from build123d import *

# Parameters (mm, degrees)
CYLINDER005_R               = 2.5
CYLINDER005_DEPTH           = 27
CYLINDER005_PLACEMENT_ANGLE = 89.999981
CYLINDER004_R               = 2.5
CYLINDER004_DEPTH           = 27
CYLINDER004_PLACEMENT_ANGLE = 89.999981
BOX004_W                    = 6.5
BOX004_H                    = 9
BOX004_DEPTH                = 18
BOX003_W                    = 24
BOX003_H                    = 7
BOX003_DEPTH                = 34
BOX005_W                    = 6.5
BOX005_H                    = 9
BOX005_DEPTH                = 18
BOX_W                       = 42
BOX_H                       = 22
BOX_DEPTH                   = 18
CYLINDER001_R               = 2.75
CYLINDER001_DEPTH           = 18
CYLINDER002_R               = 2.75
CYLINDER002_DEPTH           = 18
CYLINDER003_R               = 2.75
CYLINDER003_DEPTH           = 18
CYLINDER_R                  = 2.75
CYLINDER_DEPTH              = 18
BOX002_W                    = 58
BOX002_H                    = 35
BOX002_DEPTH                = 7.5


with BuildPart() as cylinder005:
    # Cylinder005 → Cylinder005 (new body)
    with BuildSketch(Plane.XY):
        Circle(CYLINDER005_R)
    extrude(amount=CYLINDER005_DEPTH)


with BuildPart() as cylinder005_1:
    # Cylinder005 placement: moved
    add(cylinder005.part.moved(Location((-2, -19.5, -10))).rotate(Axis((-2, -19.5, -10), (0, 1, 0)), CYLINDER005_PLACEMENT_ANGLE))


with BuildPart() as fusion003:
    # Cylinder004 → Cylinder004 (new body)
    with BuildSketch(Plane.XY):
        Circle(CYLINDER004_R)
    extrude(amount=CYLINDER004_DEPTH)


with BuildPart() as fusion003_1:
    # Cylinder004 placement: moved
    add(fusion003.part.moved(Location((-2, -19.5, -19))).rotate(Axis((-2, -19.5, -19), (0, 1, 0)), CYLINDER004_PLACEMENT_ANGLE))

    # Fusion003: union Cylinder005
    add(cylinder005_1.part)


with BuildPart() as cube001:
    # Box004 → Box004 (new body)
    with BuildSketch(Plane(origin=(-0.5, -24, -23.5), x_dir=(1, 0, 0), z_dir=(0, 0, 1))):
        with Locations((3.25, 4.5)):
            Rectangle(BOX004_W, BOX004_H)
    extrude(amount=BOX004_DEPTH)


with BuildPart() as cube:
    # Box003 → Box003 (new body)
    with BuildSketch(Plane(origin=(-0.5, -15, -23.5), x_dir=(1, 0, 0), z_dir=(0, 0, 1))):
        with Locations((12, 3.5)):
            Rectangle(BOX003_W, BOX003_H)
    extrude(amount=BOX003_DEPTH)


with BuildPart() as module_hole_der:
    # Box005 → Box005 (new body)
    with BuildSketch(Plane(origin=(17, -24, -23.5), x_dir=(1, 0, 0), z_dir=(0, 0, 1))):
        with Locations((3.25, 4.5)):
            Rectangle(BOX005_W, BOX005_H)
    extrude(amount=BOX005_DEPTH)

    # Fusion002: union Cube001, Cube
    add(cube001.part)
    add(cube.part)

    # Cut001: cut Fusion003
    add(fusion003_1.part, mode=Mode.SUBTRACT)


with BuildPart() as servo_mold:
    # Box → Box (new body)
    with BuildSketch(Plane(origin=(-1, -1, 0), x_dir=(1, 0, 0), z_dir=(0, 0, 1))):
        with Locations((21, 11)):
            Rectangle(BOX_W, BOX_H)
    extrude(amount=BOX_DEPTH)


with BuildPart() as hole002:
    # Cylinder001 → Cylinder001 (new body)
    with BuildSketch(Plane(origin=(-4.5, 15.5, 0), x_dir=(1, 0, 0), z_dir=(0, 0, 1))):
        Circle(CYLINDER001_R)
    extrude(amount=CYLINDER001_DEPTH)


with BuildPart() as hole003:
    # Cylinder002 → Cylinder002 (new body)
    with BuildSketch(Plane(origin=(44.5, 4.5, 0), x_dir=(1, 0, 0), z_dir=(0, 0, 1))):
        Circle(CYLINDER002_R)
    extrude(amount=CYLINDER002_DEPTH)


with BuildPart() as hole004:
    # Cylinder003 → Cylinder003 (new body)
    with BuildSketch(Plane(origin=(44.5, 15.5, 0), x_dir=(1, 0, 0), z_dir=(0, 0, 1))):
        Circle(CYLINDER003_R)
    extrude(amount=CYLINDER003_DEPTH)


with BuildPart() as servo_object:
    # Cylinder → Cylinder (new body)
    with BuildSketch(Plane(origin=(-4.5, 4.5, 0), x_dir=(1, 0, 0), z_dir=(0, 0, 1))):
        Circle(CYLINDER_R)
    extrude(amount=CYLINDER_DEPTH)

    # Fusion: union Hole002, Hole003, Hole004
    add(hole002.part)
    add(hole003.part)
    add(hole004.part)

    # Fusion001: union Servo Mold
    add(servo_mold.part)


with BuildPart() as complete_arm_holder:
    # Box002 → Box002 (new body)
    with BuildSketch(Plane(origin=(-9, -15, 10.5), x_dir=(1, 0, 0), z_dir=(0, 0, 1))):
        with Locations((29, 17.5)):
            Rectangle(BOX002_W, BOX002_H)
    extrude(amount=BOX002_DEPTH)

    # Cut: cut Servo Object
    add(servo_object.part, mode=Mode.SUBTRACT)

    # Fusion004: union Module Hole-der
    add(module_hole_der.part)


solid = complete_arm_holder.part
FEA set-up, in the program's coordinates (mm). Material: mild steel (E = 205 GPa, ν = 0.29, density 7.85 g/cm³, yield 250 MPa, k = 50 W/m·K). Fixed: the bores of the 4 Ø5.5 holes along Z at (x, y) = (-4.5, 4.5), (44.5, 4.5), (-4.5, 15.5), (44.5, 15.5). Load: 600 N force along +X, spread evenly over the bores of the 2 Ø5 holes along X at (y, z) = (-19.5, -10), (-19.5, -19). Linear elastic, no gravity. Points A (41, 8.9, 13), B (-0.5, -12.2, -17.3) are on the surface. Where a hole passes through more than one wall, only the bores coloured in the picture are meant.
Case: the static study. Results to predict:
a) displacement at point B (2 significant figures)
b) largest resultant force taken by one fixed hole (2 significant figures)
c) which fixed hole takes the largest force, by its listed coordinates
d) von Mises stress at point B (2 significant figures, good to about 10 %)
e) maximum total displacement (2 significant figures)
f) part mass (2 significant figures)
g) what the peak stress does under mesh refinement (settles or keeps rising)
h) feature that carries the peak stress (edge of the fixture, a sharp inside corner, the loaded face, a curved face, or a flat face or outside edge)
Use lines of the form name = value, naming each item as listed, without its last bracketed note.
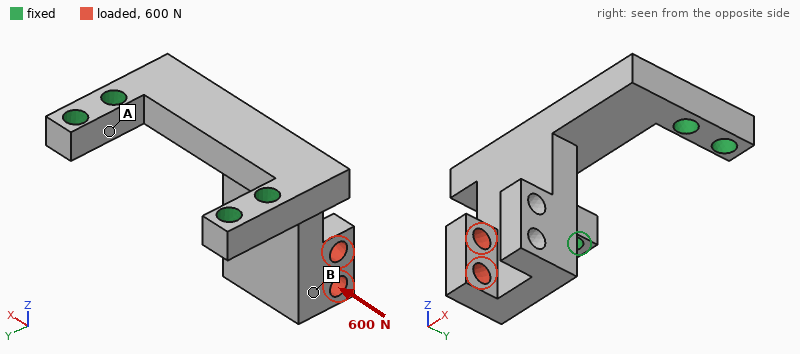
displacement at point B = 19 µm
largest resultant force taken by one fixed hole = 570 N
which fixed hole takes the largest force, by its listed coordinates = (44.5, 4.5)
von Mises stress at point B = 10 MPa
maximum total displacement = 31 µm
part mass = 120 g
what the peak stress does under mesh refinement = keeps rising
feature that carries the peak stress = edge of the fixture
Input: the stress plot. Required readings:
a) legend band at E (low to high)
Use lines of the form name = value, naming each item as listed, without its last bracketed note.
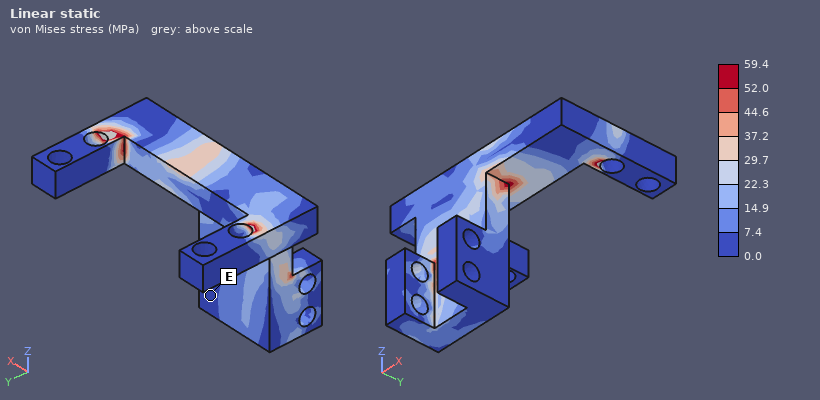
legend band at E = 0.0 to 7.4 MPa
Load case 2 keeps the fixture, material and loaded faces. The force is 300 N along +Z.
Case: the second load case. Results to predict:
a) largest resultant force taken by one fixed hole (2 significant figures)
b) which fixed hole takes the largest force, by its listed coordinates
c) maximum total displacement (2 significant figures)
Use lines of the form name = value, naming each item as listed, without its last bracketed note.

largest resultant force taken by one fixed hole = 260 N
which fixed hole takes the largest force, by its listed coordinates = (-4.5, 4.5)
maximum total displacement = 40 µm
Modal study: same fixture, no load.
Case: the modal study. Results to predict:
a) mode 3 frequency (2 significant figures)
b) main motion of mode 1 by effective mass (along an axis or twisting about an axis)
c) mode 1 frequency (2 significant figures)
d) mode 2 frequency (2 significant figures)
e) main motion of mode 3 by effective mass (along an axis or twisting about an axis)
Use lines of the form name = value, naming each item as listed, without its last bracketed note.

mode 3 frequency = 6600 Hz
main motion of mode 1 by effective mass = along Y
mode 1 frequency = 1800 Hz
mode 2 frequency = 4100 Hz
main motion of mode 3 by effective mass = along Z
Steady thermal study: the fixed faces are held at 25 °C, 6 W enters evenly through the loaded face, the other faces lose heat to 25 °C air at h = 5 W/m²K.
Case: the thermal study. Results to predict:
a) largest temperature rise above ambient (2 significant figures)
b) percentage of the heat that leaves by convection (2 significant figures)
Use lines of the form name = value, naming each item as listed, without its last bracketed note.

largest temperature rise above ambient = 43 K
percentage of the heat that leaves by convection = 9.2 %
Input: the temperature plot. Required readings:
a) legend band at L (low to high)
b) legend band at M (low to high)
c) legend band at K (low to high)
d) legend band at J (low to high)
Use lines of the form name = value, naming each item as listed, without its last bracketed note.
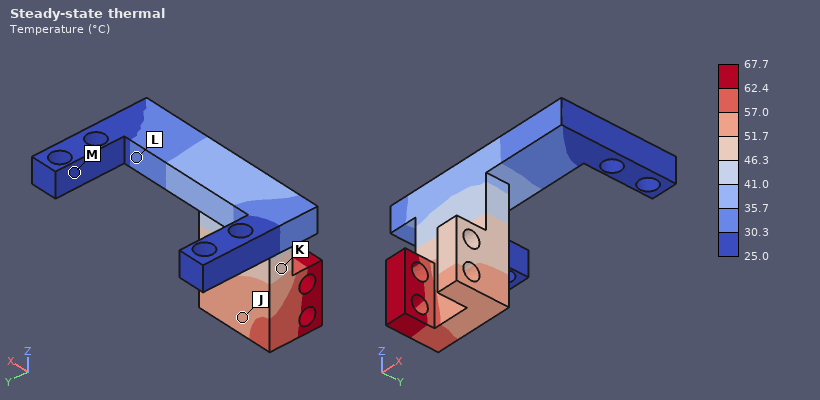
legend band at L = 30.3 to 35.7 °C
legend band at M = 25.0 to 30.3 °C
legend band at K = 46.3 to 51.7 °C
legend band at J = 51.7 to 57.0 °C
